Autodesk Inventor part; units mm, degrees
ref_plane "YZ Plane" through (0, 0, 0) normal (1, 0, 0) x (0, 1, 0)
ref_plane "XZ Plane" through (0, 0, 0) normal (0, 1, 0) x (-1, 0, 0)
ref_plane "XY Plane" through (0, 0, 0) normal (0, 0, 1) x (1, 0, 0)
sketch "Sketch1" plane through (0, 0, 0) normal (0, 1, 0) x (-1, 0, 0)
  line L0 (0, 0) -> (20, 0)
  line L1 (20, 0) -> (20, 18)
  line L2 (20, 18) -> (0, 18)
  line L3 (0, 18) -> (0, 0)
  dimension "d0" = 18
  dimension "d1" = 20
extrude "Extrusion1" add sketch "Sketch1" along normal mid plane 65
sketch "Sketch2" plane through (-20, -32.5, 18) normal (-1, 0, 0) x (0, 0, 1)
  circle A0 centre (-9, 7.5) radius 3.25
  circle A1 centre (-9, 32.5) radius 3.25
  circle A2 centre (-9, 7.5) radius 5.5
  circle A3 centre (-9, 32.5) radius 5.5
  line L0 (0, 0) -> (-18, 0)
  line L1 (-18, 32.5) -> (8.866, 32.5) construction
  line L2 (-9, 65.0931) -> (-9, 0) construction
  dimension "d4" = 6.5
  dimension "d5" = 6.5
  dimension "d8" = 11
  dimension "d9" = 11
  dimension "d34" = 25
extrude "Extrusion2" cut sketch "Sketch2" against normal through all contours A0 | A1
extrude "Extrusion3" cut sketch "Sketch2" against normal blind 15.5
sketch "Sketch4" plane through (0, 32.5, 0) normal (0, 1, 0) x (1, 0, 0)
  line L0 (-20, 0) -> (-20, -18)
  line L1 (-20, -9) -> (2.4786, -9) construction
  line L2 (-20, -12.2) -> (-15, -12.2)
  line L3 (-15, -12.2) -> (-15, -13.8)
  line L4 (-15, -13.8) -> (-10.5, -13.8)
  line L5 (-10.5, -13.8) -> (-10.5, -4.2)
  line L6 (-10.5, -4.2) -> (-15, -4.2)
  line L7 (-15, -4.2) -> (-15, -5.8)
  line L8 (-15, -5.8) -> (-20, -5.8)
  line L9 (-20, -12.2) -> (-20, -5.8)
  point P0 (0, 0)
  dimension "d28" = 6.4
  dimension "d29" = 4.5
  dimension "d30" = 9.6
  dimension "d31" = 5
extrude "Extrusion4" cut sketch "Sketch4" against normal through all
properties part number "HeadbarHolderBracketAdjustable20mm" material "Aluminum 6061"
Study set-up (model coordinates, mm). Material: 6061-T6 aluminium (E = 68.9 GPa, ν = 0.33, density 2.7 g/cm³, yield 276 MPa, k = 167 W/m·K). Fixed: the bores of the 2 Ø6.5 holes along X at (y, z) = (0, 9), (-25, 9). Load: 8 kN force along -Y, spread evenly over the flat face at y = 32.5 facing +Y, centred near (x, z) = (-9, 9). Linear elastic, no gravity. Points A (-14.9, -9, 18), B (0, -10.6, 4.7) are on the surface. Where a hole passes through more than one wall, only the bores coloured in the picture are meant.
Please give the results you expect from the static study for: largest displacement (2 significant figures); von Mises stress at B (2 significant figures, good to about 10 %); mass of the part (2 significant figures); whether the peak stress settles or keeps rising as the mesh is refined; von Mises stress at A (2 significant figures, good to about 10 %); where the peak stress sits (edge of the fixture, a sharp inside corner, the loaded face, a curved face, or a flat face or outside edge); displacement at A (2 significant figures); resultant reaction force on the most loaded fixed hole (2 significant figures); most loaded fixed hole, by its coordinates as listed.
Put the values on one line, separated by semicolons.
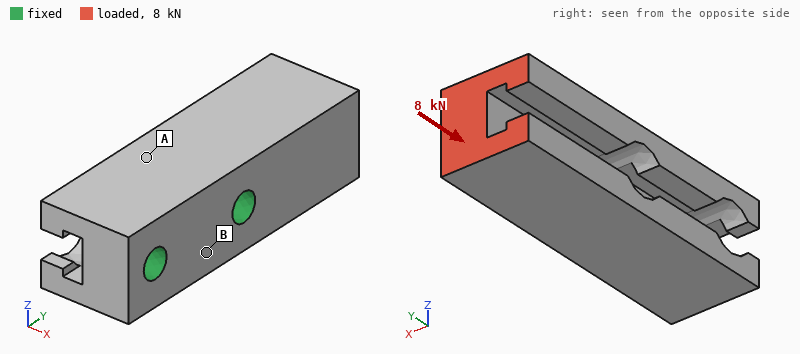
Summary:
54 µm; 13 MPa; 45 g; keeps rising; 33 MPa; edge of the fixture; 12 µm; 5.9 kN; (0, 9)
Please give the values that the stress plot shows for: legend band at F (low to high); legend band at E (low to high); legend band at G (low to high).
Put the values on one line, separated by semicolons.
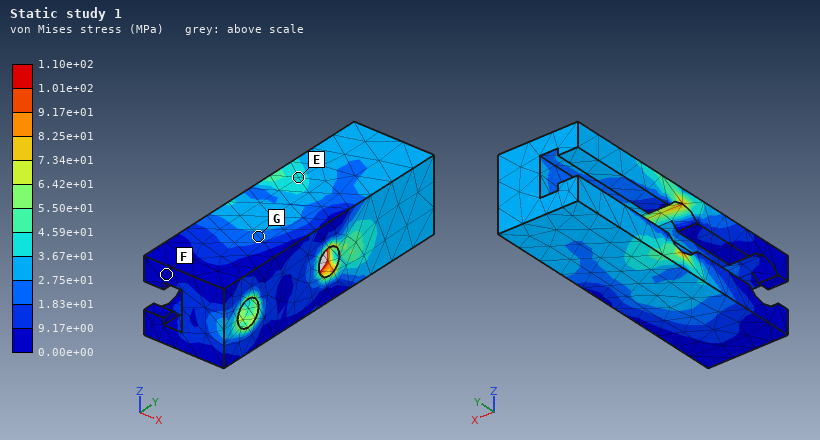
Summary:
0.00e+00 to 9.17e+00 MPa; 3.67e+01 to 4.59e+01 MPa; 1.83e+01 to 2.75e+01 MPa
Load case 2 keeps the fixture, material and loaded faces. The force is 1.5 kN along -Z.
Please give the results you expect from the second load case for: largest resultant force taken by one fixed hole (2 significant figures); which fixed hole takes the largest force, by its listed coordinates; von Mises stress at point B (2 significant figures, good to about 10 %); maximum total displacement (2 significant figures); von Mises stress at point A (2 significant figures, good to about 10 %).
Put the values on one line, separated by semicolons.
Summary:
2.7 kN; (0, 9); 22 MPa; 0.13 mm; 25 MPa
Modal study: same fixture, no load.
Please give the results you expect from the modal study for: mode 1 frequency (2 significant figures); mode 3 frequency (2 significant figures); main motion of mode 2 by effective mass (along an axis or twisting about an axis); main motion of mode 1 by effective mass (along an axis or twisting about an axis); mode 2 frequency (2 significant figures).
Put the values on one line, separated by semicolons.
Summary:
6400 Hz; 10 kHz; along X; along Z; 7800 Hz
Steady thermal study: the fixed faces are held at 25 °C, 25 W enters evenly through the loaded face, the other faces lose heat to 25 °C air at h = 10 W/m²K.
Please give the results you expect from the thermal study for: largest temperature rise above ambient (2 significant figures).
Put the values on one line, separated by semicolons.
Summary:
21 K
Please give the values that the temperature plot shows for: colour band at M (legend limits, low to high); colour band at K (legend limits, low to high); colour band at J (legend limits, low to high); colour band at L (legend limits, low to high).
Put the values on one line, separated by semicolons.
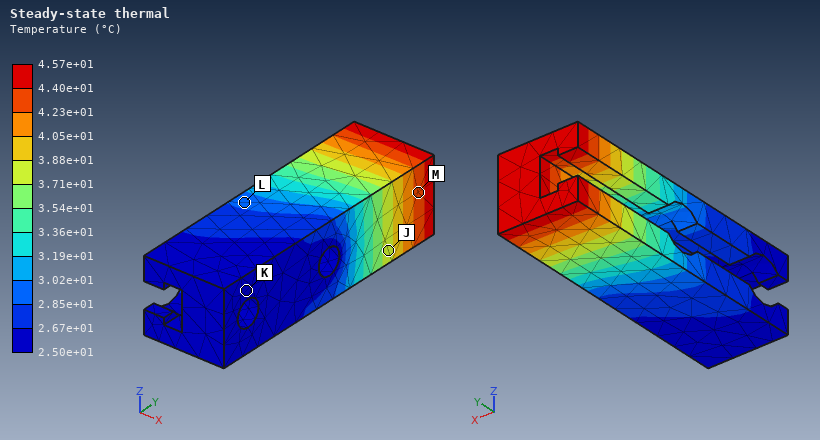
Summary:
4.23e+01 to 4.40e+01 °C; 2.50e+01 to 2.67e+01 °C; 3.71e+01 to 3.88e+01 °C; 2.85e+01 to 3.02e+01 °C
